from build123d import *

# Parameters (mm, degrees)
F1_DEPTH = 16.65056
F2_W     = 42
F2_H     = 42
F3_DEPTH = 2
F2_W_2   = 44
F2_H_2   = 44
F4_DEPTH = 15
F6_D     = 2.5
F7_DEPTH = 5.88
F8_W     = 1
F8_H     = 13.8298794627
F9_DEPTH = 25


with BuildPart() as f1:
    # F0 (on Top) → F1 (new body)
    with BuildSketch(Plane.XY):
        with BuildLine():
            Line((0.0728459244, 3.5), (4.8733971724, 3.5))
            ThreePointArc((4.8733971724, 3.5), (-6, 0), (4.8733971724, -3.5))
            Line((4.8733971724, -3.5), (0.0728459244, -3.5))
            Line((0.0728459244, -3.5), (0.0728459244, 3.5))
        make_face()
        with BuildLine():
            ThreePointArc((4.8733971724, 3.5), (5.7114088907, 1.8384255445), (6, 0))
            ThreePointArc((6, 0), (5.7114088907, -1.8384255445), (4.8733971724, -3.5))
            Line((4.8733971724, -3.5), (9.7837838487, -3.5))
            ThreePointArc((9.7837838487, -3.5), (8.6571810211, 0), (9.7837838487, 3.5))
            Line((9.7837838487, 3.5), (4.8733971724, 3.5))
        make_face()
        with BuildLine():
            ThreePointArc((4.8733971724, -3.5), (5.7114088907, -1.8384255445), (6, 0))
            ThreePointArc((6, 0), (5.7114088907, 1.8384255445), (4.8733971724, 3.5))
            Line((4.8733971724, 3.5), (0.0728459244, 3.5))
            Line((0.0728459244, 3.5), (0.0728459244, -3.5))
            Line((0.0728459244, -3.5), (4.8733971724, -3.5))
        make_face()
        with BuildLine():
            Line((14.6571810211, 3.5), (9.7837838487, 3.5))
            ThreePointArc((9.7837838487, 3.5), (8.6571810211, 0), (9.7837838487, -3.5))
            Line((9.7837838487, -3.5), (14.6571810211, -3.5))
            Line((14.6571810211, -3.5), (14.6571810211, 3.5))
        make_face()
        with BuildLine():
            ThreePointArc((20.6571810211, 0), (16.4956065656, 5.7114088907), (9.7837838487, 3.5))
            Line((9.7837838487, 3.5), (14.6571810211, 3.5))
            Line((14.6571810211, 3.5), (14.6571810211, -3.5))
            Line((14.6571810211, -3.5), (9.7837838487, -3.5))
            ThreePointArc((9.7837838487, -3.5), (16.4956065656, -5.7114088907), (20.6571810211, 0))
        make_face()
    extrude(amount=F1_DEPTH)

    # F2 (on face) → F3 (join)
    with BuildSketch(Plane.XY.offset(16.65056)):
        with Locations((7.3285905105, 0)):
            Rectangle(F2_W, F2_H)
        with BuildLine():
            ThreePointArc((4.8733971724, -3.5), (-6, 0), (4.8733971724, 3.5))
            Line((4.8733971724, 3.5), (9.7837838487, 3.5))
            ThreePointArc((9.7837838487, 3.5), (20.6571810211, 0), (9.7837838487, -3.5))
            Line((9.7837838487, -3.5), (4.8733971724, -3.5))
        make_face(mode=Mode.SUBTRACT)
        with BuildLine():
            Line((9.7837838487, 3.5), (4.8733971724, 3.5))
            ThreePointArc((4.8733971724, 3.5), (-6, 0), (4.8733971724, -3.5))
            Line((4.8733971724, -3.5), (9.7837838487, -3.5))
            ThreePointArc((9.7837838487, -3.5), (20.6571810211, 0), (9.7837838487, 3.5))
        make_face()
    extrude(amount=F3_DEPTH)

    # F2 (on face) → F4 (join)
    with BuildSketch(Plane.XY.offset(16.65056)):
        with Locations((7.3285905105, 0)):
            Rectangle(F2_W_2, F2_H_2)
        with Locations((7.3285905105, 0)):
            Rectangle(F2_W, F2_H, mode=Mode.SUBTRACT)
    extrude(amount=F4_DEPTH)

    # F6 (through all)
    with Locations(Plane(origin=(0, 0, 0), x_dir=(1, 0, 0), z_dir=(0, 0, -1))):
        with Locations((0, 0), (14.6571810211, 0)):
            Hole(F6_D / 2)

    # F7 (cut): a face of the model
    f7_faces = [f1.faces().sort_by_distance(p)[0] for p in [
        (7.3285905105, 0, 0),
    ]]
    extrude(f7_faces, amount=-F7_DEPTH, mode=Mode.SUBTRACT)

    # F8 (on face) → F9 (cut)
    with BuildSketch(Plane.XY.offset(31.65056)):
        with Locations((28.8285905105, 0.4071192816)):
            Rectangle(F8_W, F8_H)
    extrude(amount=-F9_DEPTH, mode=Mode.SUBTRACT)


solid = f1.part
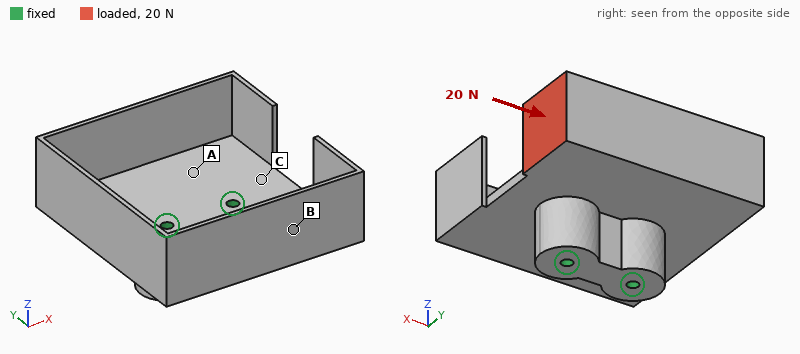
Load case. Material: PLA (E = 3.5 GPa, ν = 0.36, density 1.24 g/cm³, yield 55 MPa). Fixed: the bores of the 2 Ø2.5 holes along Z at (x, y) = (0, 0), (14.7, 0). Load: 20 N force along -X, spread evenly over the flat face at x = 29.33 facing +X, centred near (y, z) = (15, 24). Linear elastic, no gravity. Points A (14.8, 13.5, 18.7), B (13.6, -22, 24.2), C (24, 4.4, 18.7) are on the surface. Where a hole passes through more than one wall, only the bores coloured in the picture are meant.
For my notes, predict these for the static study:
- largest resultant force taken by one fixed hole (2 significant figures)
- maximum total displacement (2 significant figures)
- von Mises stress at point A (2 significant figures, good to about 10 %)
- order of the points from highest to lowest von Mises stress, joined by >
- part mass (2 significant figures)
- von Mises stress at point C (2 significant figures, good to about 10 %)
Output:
22 N
0.69 mm
2.2 MPa
C > A > B
10 g
3.4 MPa
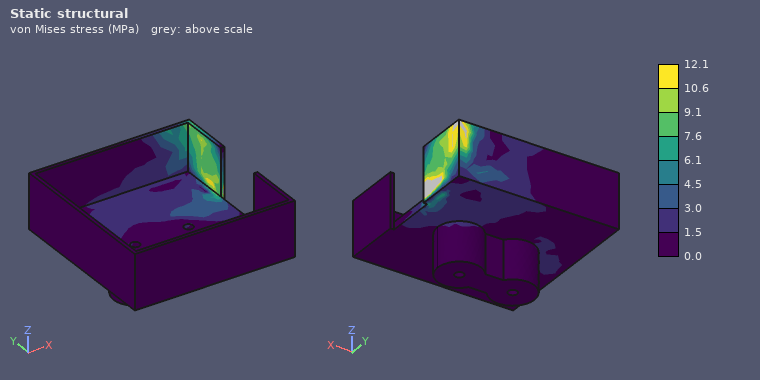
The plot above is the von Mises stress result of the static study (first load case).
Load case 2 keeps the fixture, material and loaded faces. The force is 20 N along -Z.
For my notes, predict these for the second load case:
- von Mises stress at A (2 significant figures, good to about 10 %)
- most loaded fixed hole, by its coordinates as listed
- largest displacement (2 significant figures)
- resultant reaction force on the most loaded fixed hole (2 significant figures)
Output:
6.1 MPa
(14.7, 0)
0.72 mm
27 N
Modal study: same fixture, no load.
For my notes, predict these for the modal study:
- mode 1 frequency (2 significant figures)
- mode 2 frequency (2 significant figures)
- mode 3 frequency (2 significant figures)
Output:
930 Hz
940 Hz
960 Hz
